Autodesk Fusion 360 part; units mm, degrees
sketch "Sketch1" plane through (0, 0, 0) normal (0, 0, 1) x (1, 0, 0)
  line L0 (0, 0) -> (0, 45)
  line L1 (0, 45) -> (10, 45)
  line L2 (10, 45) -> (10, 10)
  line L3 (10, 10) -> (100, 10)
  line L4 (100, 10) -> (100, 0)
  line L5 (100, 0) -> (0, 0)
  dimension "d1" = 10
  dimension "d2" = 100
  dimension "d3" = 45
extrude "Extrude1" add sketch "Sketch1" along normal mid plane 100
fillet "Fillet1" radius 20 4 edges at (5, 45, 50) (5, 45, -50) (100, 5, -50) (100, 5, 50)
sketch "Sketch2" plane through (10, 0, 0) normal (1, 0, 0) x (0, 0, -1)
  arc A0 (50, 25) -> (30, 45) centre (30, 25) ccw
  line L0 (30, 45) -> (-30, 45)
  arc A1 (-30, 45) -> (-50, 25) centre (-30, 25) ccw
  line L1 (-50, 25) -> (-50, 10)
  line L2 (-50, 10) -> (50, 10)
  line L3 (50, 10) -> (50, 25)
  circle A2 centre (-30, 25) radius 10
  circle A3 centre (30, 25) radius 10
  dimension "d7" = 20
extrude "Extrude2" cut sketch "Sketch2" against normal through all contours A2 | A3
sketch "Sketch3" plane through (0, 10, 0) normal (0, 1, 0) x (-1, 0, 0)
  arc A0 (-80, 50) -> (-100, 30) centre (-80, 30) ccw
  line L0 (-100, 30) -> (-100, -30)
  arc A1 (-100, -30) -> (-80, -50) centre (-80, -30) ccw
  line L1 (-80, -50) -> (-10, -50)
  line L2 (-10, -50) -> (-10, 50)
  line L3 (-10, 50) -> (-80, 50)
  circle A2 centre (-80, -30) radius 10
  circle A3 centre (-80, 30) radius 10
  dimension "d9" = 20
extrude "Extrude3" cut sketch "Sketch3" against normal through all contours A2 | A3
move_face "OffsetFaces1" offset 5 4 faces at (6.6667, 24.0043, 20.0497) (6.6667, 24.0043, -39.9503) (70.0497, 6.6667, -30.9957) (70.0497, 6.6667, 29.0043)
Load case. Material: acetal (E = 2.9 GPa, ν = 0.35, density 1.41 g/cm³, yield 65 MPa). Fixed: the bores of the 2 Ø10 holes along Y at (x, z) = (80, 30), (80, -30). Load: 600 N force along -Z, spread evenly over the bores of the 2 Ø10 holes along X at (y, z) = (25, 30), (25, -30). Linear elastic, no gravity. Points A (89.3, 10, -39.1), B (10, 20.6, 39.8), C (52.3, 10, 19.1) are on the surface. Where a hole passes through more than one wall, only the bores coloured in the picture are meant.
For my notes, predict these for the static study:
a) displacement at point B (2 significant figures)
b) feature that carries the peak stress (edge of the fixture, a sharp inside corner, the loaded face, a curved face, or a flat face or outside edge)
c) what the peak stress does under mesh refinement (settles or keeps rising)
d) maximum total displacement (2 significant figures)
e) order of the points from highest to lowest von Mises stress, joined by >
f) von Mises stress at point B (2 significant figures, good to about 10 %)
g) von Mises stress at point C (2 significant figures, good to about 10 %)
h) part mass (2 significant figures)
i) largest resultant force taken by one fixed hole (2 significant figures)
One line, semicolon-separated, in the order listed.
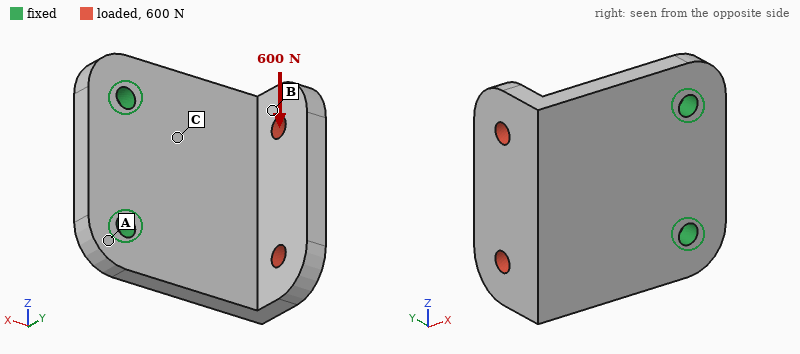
0.64 mm; edge of the fixture; keeps rising; 0.89 mm; C > B > A; 3.3 MPa; 5.5 MPa; 180 g; 760 N
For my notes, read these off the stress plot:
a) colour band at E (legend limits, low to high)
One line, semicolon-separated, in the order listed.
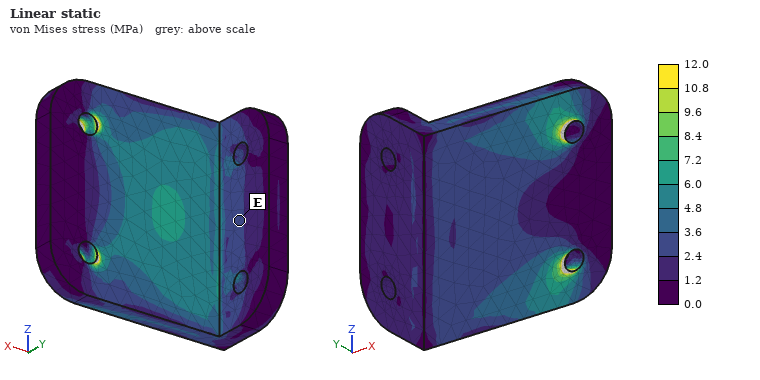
2.4 to 3.6 MPa
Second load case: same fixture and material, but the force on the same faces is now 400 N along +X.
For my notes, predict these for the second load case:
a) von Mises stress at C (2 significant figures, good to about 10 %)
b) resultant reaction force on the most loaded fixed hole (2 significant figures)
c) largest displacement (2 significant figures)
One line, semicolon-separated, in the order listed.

4.7 MPa; 200 N; 1.4 mm
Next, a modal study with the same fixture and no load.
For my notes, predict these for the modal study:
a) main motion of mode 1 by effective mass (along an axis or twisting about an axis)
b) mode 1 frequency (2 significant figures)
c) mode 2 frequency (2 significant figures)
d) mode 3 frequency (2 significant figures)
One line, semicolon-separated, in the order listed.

along Y; 220 Hz; 470 Hz; 910 Hz
